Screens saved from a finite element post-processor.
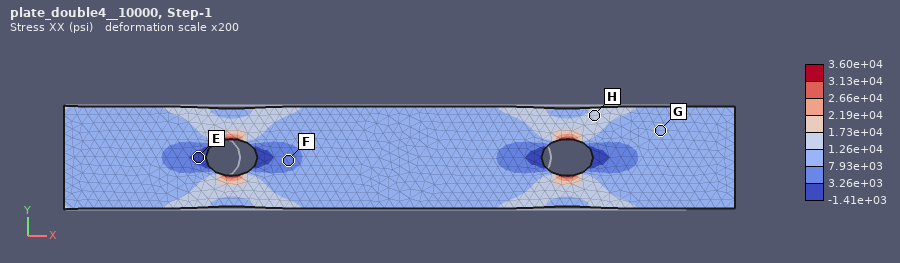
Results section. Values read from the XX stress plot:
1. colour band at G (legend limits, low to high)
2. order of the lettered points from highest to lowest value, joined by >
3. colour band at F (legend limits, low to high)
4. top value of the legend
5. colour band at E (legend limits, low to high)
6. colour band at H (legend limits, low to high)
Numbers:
7.93e+03 to 1.26e+04 psi
H > G > F > E
3.26e+03 to 7.93e+03 psi
3.60e+04 psi
-1.41e+03 to 3.26e+03 psi
1.26e+04 to 1.73e+04 psi
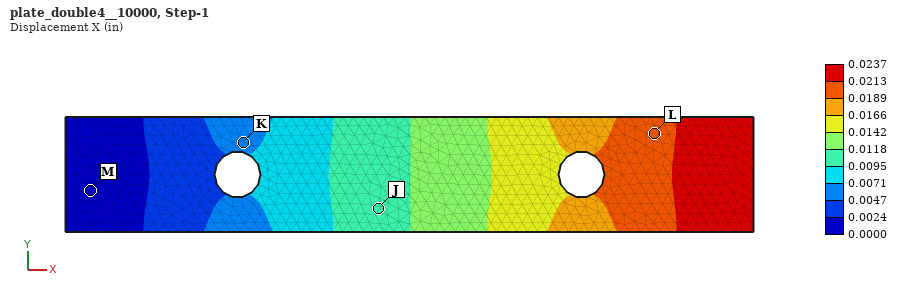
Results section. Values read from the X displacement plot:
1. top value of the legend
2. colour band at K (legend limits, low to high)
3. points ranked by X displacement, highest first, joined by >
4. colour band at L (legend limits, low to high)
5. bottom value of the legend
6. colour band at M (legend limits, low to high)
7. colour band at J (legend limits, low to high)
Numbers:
0.0237 in
0.0047 to 0.0071 in
L > J > K > M
0.0189 to 0.0213 in
0.0000 in
0.0000 to 0.0024 in
0.0095 to 0.0118 in
